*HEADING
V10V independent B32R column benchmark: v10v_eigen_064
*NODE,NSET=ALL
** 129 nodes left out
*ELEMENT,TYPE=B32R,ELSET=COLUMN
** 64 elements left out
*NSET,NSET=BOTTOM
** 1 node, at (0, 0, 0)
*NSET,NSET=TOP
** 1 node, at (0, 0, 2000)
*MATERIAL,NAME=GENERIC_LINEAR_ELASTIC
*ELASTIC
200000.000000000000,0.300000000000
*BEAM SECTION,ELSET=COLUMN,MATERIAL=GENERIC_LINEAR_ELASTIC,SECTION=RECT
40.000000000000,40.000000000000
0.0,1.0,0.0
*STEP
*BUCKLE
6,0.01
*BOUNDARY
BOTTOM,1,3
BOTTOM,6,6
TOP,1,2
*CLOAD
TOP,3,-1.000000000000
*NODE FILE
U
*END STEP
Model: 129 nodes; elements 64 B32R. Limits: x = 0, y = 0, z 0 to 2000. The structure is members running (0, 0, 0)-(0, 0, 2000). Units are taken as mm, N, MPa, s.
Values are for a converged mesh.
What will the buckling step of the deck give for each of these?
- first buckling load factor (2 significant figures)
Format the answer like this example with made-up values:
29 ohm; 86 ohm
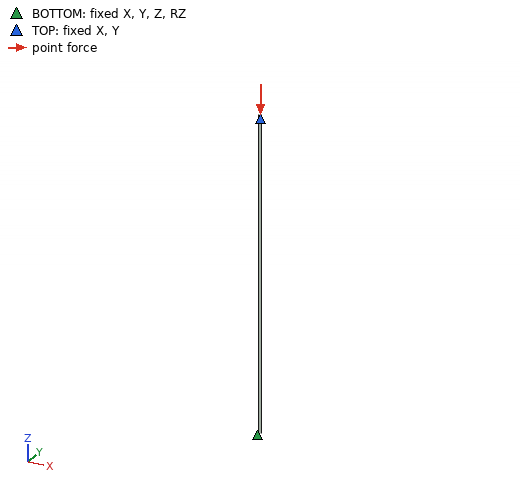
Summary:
1.1e+05
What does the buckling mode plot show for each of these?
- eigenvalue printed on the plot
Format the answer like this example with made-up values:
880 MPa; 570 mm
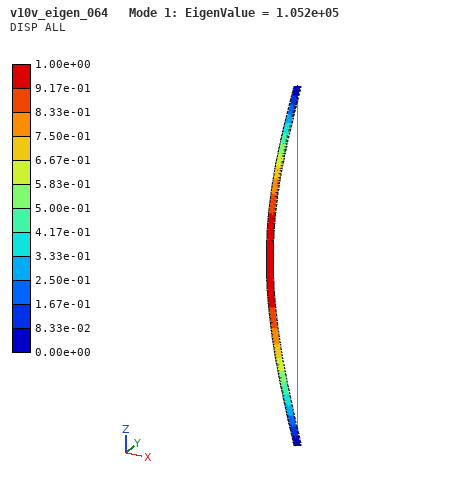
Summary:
1.052e+05
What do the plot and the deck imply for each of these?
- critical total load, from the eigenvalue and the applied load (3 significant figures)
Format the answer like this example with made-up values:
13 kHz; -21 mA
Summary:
1.05e+05 N
